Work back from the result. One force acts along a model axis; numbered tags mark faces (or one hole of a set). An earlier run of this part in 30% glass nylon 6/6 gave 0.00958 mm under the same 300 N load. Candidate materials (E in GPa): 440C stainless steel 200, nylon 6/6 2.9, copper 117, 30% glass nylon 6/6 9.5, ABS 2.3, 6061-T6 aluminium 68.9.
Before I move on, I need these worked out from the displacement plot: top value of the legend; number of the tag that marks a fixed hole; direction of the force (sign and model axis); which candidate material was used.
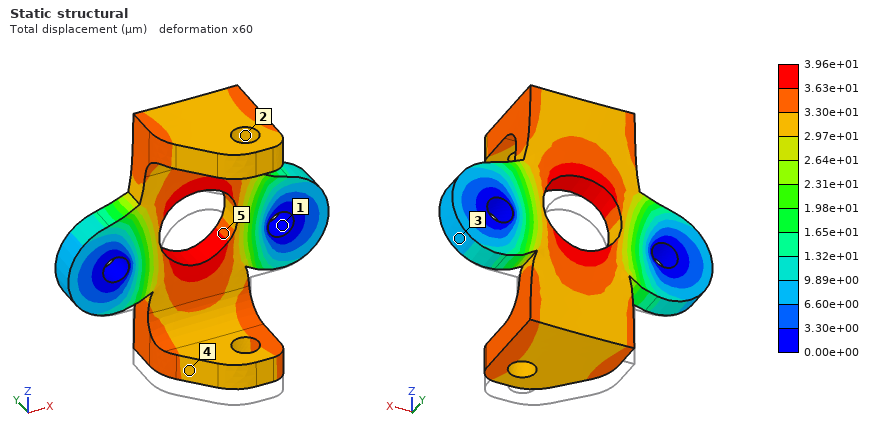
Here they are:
3.96e+01 µm
1
+Z
ABS
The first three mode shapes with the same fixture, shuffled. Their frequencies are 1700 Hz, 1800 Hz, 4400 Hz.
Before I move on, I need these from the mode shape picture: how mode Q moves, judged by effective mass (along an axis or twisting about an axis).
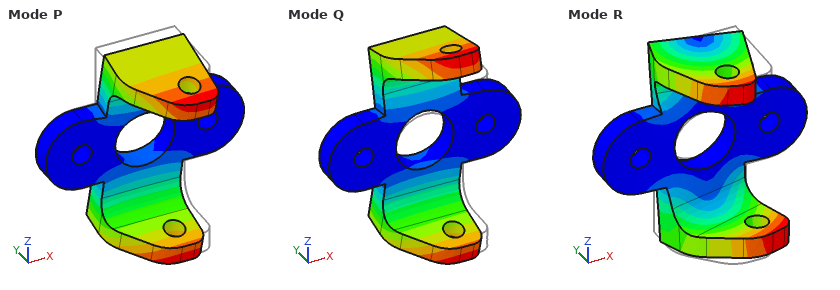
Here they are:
along Y
